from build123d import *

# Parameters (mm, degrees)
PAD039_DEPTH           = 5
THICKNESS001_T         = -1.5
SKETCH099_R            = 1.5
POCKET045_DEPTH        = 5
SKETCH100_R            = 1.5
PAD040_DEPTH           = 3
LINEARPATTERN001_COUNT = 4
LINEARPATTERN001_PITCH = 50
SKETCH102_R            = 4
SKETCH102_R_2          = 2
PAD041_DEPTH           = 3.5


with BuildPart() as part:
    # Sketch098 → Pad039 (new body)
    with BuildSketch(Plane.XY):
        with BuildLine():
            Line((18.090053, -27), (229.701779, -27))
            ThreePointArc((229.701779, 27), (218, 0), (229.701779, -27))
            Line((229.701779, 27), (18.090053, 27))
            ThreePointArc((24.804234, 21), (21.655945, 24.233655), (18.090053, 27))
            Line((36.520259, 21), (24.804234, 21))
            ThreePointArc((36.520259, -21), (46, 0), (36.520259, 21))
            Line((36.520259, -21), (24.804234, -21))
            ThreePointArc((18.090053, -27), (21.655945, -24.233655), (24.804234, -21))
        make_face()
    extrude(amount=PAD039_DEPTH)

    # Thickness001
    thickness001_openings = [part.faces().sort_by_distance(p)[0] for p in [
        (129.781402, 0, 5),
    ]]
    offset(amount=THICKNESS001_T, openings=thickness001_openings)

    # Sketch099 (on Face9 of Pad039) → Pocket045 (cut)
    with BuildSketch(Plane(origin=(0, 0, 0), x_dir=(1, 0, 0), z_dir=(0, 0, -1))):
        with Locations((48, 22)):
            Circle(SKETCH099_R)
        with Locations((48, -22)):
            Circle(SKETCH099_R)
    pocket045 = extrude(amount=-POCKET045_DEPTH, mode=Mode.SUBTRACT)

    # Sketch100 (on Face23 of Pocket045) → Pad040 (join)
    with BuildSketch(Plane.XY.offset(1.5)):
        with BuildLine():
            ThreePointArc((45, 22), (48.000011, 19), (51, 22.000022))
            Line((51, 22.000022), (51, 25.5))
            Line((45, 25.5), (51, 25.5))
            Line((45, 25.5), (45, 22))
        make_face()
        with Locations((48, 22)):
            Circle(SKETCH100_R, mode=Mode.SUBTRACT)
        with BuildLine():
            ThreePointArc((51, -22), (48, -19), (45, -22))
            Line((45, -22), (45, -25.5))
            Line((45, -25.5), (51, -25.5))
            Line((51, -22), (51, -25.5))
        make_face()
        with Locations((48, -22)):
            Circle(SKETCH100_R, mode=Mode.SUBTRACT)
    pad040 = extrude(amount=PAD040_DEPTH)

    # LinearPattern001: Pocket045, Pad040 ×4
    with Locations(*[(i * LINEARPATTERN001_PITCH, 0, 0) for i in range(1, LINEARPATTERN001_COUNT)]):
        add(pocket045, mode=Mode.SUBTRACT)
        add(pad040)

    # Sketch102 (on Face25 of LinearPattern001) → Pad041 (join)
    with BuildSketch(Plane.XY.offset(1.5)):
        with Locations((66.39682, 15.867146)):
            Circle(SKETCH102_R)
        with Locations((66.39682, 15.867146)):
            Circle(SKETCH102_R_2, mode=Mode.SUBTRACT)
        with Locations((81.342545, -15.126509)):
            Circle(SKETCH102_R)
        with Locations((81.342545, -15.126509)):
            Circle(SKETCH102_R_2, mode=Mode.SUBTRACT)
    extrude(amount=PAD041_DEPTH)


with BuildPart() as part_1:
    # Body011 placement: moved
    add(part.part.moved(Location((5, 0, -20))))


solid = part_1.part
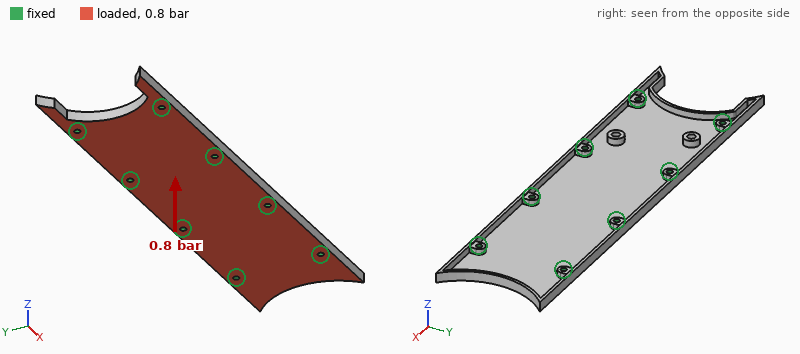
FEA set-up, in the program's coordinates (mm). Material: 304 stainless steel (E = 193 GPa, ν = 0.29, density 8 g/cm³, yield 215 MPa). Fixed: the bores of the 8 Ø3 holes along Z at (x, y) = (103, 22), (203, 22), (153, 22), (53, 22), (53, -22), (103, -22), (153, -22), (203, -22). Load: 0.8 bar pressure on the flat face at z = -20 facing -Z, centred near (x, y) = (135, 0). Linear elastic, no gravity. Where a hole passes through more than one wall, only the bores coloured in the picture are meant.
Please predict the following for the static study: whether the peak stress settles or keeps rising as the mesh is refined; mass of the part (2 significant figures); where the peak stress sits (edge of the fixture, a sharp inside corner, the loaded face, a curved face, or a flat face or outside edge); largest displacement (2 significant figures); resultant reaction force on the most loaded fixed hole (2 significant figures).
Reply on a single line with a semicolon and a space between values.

keeps rising; 150 g; edge of the fixture; 30 µm; 120 N
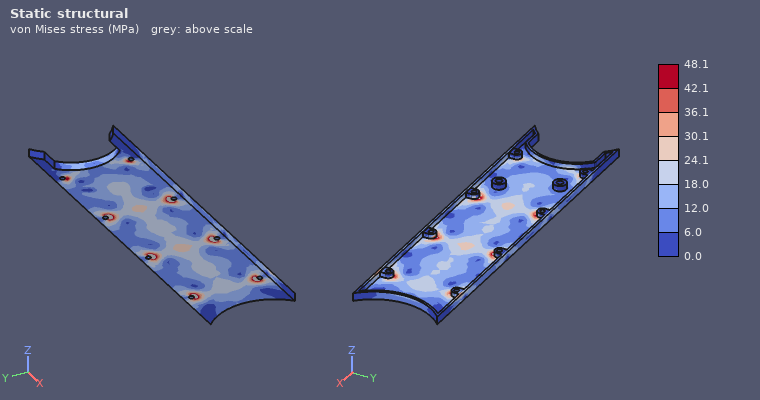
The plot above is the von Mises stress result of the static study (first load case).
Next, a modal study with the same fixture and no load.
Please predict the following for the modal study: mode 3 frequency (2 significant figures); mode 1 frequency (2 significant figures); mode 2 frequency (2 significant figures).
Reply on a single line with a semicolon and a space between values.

2900 Hz; 2600 Hz; 2900 Hz
